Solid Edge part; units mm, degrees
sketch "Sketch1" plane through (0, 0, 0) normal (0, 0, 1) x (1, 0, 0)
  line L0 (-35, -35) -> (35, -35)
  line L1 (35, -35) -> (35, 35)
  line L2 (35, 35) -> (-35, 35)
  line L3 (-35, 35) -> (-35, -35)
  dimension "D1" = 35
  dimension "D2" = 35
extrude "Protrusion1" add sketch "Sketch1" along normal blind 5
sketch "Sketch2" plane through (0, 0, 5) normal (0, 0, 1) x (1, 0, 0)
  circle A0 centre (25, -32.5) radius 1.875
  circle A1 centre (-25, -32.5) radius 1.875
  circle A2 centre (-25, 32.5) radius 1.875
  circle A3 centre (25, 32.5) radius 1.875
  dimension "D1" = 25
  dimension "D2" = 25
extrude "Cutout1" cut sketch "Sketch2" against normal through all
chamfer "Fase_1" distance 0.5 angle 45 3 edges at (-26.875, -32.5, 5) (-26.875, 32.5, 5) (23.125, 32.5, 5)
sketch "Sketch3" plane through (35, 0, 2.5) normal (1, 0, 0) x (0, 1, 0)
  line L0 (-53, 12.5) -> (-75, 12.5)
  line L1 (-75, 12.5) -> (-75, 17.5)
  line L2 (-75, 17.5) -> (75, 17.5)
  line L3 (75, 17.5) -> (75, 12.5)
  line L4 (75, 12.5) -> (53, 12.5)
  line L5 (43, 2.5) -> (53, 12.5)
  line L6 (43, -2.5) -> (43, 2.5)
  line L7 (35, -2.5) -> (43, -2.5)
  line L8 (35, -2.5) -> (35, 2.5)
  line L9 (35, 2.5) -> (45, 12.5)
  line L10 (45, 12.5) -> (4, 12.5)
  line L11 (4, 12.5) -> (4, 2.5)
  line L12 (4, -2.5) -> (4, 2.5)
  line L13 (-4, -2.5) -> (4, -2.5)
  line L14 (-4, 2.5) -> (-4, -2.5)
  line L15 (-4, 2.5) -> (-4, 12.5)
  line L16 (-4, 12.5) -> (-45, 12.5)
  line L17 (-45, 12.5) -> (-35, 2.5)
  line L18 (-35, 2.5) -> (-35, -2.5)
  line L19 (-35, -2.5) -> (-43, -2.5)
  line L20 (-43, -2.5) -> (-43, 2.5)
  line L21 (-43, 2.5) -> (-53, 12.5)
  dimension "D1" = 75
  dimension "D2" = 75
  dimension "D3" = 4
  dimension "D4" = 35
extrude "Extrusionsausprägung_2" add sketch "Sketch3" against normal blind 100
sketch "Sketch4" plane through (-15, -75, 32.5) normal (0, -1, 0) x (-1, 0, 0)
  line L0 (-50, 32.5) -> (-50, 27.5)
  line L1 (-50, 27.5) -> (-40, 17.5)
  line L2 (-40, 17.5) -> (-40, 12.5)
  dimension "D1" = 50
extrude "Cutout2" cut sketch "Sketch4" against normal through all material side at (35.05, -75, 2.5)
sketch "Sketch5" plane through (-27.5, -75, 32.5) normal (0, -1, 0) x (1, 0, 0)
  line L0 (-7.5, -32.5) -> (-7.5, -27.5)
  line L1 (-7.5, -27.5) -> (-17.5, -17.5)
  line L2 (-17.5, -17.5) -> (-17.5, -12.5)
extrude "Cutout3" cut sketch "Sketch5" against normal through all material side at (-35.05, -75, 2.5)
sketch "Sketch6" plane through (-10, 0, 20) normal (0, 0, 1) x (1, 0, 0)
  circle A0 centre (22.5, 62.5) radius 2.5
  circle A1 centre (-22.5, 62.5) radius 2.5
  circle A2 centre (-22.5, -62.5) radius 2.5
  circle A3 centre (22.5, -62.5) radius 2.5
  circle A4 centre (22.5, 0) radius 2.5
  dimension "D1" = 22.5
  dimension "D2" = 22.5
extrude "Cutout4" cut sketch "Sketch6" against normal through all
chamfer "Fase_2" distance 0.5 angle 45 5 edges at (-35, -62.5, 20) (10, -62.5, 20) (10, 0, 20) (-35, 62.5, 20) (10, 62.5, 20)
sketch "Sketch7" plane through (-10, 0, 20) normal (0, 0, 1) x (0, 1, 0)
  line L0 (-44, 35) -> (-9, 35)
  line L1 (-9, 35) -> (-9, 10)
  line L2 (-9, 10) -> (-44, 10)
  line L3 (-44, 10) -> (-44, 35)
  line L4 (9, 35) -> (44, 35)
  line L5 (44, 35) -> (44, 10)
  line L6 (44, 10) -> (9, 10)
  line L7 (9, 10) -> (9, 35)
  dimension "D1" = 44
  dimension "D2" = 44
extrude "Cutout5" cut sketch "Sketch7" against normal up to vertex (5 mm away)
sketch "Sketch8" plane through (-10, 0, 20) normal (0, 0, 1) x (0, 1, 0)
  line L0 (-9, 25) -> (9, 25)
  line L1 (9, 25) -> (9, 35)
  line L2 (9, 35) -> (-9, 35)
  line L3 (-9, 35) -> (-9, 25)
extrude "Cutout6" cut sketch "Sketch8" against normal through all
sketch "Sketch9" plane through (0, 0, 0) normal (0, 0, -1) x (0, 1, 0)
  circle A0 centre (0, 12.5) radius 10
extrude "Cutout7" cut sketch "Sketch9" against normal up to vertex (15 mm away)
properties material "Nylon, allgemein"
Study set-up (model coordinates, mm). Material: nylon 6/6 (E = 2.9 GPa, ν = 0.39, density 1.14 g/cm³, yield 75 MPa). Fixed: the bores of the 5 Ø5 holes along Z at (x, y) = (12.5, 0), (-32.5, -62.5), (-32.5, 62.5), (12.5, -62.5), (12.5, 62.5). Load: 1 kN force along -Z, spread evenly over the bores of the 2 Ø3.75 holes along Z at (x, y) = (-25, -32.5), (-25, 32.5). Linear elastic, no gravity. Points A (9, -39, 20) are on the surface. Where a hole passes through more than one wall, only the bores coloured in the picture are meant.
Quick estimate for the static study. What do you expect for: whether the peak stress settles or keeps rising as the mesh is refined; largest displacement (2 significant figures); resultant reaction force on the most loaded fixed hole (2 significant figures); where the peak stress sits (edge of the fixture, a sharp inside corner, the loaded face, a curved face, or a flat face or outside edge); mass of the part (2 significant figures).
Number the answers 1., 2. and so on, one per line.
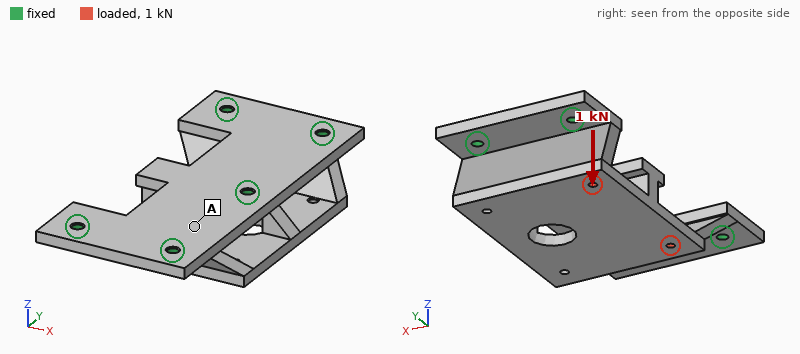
1. keeps rising
2. 0.37 mm
3. 610 N
4. edge of the fixture
5. 97 g
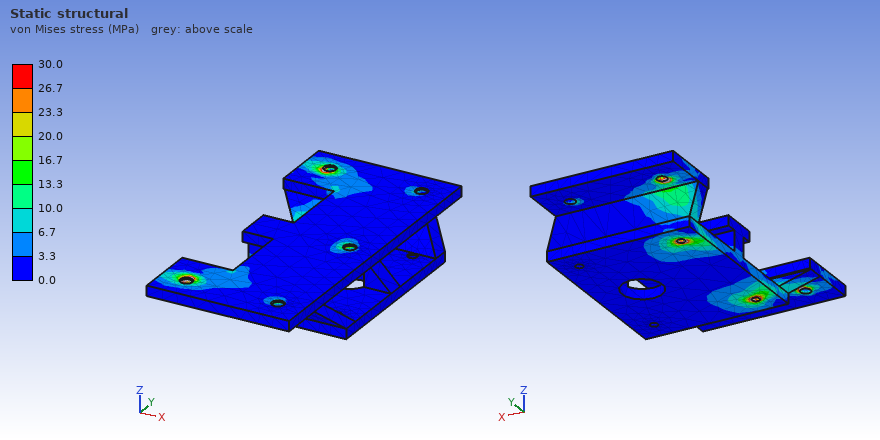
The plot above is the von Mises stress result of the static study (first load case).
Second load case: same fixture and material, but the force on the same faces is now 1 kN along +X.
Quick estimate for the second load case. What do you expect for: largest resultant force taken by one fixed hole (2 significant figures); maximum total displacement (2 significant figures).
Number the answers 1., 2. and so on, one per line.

1. 350 N
2. 0.21 mm
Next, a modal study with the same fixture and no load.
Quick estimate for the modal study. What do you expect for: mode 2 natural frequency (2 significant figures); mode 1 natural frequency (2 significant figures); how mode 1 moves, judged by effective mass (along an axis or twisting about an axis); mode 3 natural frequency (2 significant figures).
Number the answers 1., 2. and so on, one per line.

1. 1800 Hz
2. 1400 Hz
3. along Z
4. 1800 Hz
